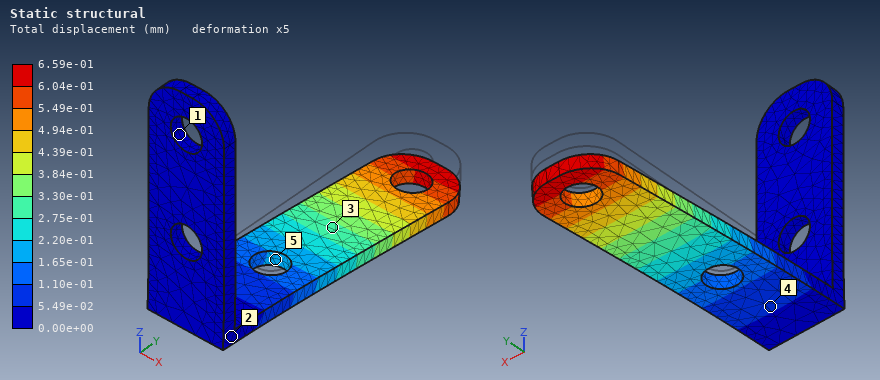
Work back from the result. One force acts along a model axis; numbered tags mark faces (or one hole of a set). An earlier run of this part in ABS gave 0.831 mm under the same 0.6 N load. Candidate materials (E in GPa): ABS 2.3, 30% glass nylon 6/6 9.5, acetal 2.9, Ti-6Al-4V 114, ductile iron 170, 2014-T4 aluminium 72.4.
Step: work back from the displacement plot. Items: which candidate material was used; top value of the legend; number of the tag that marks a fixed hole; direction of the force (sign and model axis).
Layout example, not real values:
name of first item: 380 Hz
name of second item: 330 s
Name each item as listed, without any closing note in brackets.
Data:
which candidate material was used: acetal
top value of the legend: 6.59e-01 mm
number of the tag that marks a fixed hole: 1
direction of the force: -Z
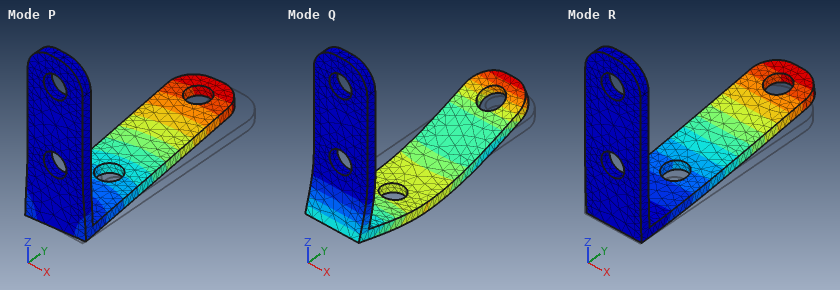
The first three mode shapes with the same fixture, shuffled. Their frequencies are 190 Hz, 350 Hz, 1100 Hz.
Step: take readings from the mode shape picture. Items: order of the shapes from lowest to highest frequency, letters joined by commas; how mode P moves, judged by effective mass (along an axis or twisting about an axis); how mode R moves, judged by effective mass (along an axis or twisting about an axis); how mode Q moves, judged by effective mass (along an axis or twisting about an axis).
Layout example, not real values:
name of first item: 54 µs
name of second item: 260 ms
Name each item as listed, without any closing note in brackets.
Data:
order of the shapes from lowest to highest frequency, letters joined by commas: R, P, Q
how mode P moves, judged by effective mass: along X
how mode R moves, judged by effective mass: along Z
how mode Q moves, judged by effective mass: along Y
